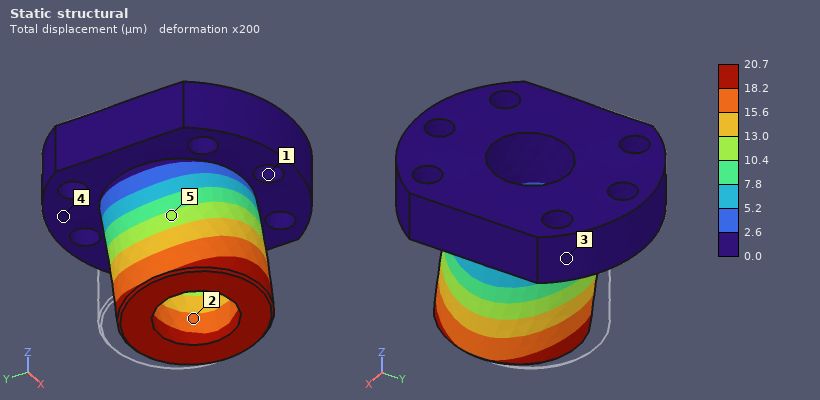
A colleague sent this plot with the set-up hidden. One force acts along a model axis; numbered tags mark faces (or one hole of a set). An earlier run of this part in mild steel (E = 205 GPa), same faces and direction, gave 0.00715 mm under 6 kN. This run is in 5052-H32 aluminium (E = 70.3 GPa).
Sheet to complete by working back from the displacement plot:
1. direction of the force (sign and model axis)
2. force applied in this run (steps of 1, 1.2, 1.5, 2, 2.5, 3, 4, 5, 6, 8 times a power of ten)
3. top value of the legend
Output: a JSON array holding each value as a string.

["-Y", "6 kN", "20.7 µm"]
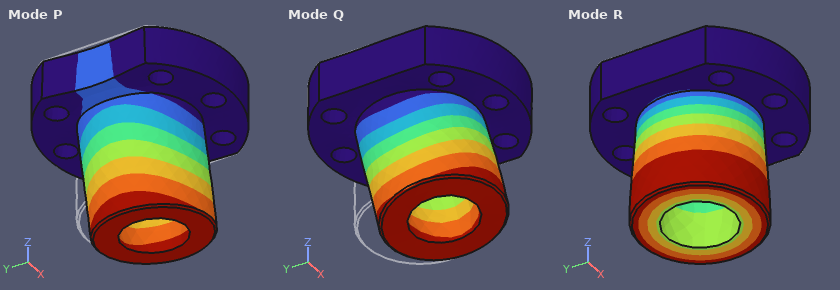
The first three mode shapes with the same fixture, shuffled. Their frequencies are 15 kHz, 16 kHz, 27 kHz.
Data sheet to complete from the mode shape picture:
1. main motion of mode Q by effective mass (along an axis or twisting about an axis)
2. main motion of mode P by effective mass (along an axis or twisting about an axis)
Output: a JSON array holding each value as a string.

["along Y", "along X"]
